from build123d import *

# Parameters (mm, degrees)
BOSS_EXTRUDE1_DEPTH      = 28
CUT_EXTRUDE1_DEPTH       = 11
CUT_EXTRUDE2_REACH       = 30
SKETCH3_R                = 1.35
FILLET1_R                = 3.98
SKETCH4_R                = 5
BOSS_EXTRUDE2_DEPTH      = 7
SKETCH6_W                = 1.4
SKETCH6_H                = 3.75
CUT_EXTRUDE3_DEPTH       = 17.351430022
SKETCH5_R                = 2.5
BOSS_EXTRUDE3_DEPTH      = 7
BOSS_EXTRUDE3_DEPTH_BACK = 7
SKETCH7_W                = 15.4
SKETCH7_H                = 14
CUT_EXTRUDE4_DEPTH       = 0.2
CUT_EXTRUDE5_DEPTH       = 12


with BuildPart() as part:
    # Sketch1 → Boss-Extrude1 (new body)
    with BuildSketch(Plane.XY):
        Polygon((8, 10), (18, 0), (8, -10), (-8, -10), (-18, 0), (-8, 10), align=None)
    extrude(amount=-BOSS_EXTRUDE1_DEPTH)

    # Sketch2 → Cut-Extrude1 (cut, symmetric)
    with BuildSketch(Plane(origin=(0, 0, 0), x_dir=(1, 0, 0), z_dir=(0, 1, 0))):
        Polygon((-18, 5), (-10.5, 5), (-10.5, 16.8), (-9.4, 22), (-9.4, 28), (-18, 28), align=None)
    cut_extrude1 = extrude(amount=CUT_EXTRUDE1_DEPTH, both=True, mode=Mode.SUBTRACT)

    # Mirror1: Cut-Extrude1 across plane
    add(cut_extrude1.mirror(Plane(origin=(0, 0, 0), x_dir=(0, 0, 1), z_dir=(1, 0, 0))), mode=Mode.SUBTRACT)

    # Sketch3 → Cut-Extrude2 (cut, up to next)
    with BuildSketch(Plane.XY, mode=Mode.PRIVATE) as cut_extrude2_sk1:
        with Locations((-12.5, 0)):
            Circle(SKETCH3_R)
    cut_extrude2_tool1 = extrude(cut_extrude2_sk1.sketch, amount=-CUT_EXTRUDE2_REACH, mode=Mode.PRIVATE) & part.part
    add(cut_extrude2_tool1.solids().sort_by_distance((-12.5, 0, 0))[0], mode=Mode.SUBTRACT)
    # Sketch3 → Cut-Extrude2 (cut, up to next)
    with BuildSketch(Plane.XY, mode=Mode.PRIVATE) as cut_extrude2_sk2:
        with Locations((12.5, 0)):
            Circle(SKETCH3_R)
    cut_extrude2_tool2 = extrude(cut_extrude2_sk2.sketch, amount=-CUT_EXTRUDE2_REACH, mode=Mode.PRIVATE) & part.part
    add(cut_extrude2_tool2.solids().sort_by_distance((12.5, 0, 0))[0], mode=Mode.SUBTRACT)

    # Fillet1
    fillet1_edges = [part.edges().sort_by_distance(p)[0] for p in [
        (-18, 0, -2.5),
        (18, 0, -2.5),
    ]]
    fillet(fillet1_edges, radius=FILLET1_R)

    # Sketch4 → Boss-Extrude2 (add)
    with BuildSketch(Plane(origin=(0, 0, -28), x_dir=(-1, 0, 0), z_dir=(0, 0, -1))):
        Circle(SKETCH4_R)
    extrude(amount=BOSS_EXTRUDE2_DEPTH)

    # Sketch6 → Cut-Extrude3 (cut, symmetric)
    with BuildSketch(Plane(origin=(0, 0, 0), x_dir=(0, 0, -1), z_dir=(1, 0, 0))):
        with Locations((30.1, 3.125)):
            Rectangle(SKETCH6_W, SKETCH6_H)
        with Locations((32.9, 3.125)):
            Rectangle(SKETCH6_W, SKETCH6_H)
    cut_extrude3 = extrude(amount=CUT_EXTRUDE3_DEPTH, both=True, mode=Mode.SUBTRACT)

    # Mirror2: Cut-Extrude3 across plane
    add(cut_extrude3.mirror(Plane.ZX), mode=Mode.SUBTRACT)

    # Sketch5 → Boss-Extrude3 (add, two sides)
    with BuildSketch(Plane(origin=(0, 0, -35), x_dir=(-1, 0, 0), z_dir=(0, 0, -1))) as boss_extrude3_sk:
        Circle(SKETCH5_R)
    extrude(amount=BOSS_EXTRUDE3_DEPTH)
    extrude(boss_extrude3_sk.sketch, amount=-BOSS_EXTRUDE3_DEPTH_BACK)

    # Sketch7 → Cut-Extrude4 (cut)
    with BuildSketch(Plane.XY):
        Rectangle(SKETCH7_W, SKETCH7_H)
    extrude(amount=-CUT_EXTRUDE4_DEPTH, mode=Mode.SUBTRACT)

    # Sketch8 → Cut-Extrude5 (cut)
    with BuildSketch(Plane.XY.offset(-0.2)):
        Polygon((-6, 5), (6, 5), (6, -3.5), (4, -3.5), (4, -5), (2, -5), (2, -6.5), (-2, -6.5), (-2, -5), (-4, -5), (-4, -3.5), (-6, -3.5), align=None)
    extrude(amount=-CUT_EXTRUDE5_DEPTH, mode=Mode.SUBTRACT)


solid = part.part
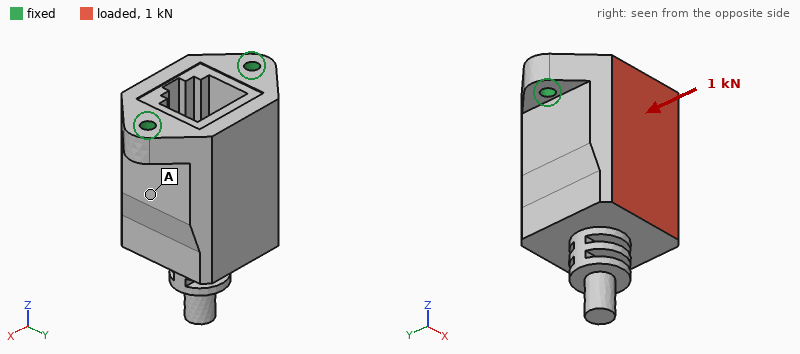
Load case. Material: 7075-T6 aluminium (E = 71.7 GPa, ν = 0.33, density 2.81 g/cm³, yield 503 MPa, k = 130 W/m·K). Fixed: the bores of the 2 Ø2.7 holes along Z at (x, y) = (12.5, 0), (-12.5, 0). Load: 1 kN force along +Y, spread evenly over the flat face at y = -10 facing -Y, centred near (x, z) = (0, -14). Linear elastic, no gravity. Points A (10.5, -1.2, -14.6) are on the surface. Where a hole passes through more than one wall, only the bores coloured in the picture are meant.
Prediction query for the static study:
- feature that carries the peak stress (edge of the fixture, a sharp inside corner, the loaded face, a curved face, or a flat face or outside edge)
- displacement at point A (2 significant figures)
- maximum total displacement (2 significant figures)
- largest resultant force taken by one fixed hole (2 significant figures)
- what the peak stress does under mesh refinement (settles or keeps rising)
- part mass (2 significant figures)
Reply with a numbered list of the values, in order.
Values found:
1. edge of the fixture
2. 29 µm
3. 91 µm
4. 500 N
5. keeps rising
6. 30 g
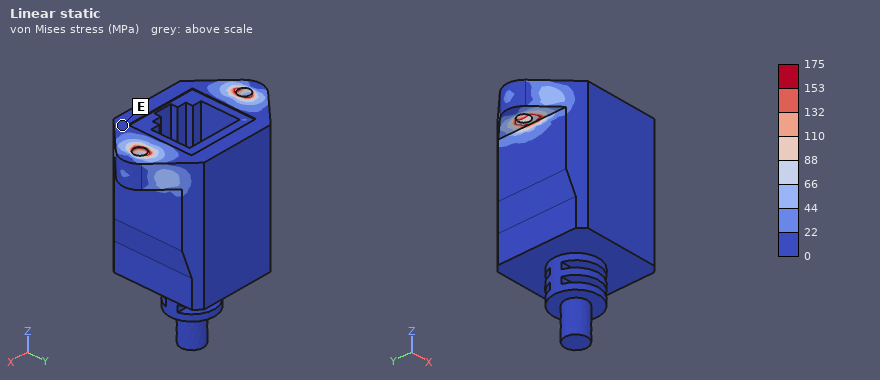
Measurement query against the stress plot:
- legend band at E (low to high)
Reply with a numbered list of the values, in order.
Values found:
1. 0 to 22 MPa
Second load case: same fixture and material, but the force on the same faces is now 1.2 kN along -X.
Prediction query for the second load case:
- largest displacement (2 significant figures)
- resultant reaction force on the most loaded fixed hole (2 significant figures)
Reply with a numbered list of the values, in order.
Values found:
1. 13 µm
2. 960 N
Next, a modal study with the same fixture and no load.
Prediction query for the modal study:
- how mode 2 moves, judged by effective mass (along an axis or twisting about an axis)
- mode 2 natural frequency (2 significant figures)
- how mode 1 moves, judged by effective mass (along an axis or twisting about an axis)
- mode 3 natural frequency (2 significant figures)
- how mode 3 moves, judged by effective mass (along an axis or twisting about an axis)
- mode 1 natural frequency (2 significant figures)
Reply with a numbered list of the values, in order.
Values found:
1. along X
2. 11 kHz
3. along Y
4. 18 kHz
5. along Z
6. 3900 Hz
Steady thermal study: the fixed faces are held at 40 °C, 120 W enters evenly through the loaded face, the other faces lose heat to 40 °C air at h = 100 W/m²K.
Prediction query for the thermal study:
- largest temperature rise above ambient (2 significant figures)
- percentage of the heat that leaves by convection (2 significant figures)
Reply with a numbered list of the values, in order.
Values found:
1. 74 K
2. 14 %
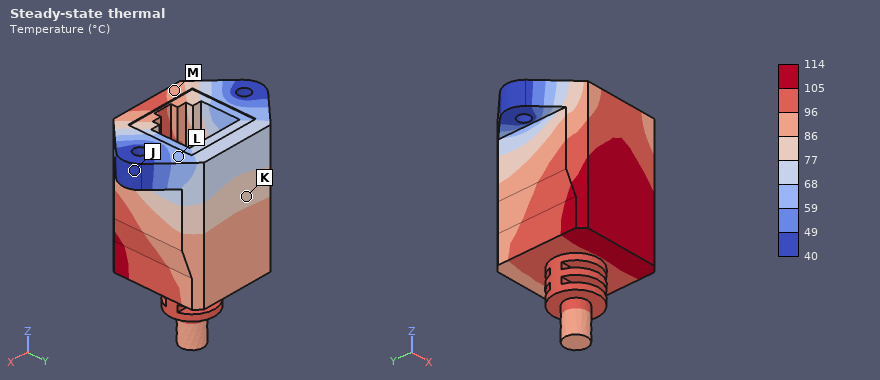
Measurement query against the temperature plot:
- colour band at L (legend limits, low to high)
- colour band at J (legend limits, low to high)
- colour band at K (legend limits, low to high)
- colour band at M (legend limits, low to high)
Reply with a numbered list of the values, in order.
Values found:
1. 59 to 68 °C
2. 40 to 49 °C
3. 77 to 86 °C
4. 86 to 96 °C
